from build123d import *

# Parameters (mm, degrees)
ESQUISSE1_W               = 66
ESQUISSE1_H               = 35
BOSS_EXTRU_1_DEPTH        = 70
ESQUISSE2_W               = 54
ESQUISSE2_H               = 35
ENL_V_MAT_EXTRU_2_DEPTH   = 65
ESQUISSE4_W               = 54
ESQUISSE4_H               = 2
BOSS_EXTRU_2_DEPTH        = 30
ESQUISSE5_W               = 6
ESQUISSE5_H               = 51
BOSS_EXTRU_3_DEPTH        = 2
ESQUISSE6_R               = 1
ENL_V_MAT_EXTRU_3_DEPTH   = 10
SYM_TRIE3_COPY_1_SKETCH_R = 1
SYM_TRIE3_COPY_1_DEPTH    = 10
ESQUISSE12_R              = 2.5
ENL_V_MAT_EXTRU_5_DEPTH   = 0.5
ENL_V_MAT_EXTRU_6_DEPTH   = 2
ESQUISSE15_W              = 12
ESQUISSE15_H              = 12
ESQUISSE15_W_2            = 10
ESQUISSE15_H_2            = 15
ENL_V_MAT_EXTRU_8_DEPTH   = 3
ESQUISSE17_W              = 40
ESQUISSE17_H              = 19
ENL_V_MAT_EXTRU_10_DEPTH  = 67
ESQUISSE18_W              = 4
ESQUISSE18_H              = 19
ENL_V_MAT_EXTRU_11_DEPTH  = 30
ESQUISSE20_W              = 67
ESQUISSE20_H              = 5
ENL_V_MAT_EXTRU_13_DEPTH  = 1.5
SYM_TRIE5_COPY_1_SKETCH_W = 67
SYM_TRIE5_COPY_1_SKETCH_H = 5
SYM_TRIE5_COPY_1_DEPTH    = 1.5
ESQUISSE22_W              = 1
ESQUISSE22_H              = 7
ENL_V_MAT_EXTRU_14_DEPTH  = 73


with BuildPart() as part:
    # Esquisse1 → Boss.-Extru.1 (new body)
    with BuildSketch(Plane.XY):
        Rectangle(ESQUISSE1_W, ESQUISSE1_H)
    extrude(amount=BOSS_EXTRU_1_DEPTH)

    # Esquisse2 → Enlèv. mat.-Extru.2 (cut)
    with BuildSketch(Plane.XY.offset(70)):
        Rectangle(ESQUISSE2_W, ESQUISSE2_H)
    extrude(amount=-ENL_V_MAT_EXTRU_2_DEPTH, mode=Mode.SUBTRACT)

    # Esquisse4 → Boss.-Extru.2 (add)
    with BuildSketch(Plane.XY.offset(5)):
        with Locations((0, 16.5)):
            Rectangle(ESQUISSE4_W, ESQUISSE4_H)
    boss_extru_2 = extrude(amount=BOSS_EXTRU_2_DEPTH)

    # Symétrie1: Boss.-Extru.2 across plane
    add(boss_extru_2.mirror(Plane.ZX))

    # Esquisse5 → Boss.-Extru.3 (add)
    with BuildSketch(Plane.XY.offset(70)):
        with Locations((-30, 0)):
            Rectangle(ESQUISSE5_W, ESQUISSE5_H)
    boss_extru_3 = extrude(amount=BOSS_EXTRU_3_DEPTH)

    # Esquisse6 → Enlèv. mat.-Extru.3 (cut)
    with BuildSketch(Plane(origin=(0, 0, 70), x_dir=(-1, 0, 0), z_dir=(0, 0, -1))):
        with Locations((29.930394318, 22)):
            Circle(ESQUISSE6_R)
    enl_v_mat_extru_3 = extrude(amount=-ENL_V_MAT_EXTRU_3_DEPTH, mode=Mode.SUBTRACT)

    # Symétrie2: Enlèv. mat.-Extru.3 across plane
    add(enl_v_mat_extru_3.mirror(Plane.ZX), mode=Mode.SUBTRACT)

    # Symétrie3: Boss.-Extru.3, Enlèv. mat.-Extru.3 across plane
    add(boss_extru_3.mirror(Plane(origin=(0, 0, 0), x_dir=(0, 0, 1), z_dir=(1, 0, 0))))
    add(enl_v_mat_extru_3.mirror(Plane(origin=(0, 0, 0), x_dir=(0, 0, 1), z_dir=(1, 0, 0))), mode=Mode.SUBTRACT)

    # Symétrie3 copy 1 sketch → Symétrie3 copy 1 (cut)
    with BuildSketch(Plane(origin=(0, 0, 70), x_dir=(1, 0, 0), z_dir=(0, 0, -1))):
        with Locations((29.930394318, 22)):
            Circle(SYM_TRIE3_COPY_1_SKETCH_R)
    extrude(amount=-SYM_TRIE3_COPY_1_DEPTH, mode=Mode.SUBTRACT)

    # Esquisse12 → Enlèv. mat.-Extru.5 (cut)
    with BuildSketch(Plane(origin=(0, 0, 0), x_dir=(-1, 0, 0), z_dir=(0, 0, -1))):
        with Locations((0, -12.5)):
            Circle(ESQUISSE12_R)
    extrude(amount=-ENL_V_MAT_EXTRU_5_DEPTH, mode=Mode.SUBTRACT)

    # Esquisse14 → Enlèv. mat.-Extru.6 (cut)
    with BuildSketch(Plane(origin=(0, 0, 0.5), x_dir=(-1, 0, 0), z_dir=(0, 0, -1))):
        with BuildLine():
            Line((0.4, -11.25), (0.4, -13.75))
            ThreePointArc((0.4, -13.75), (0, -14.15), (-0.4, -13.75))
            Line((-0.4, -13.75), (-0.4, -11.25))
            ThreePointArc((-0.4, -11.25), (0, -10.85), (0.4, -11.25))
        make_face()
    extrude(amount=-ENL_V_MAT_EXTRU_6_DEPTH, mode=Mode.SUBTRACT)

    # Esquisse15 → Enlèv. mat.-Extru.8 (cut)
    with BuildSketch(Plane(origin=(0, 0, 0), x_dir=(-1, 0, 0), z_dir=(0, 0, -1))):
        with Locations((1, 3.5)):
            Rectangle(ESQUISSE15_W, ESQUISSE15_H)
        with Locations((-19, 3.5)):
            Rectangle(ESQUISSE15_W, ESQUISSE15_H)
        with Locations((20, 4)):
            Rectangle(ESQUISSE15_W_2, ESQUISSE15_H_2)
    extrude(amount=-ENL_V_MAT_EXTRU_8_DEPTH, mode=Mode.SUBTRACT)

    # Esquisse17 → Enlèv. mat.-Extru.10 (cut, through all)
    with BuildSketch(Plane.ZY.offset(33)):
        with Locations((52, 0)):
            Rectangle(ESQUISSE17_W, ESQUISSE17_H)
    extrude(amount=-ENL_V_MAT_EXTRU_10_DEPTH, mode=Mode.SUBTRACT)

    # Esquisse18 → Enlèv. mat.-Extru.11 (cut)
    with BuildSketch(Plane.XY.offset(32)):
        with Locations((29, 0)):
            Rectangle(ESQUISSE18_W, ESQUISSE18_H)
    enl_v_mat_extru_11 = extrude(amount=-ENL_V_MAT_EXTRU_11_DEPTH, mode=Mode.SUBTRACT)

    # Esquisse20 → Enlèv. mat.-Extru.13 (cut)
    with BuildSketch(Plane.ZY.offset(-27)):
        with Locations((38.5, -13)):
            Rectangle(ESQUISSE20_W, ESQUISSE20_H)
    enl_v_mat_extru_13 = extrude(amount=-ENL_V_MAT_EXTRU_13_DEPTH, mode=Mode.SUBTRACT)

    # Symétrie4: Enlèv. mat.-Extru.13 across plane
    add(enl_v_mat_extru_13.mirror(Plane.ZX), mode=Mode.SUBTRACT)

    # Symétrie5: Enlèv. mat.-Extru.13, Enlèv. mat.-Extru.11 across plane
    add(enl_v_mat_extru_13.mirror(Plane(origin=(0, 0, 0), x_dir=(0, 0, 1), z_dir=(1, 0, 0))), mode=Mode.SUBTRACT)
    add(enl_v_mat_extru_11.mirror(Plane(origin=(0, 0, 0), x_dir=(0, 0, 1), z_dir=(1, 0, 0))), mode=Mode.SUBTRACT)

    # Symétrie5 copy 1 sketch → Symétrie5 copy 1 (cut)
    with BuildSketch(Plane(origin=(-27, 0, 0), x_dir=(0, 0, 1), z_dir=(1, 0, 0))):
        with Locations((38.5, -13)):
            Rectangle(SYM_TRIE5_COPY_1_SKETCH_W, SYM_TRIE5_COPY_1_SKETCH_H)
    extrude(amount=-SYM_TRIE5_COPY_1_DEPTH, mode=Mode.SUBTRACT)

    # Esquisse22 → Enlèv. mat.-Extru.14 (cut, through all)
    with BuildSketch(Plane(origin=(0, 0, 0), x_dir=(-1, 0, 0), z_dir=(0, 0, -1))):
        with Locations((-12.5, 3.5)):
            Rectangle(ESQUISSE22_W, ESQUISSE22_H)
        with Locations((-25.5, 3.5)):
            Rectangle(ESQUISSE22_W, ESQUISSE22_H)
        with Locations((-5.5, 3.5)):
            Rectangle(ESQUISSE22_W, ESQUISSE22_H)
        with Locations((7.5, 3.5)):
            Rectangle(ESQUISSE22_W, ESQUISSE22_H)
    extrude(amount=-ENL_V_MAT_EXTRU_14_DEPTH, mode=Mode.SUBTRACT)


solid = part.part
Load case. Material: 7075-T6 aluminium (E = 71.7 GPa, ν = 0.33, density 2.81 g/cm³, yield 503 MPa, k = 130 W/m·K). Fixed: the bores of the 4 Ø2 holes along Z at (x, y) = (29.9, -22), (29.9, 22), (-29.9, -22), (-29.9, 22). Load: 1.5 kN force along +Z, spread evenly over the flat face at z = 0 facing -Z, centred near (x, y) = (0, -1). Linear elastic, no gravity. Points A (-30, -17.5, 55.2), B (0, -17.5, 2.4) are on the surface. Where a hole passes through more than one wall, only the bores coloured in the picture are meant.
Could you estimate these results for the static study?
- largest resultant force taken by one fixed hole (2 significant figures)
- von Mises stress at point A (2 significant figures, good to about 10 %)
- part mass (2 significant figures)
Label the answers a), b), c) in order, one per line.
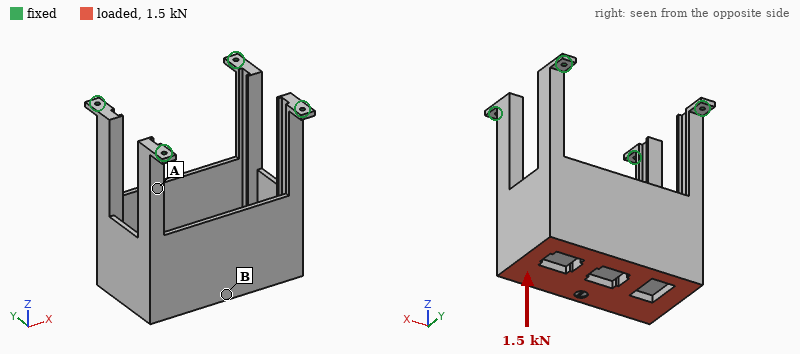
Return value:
a) 400 N
b) 27 MPa
c) 83 g
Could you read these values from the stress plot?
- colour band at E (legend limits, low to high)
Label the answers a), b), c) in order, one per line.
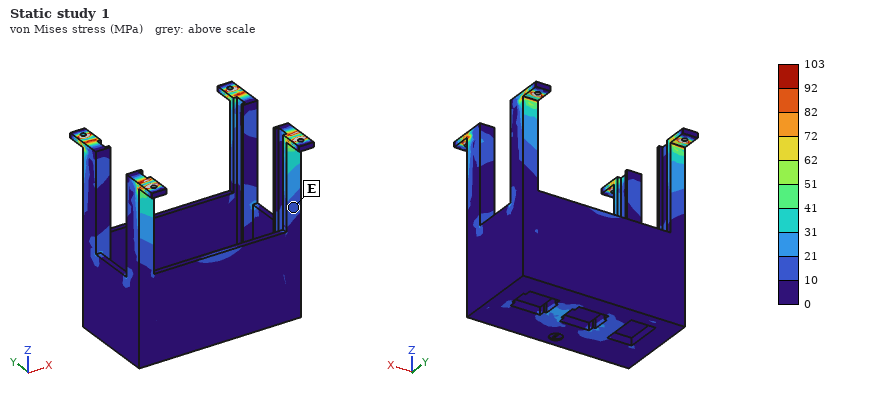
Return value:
a) 10 to 21 MPa
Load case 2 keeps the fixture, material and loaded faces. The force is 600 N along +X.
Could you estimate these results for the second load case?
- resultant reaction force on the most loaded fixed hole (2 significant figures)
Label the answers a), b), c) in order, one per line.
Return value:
a) 360 N
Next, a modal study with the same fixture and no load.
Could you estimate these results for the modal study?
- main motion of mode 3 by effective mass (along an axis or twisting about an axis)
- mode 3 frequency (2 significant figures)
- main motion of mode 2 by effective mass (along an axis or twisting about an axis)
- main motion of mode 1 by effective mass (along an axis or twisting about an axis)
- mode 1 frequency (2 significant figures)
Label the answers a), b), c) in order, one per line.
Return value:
a) twisting about Z
b) 1500 Hz
c) along Y
d) along X
e) 690 Hz
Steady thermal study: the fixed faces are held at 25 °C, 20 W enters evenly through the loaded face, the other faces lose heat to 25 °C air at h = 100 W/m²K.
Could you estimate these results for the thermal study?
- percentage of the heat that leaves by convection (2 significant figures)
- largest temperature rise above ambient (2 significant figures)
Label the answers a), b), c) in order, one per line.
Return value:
a) 90 %
b) 14 K
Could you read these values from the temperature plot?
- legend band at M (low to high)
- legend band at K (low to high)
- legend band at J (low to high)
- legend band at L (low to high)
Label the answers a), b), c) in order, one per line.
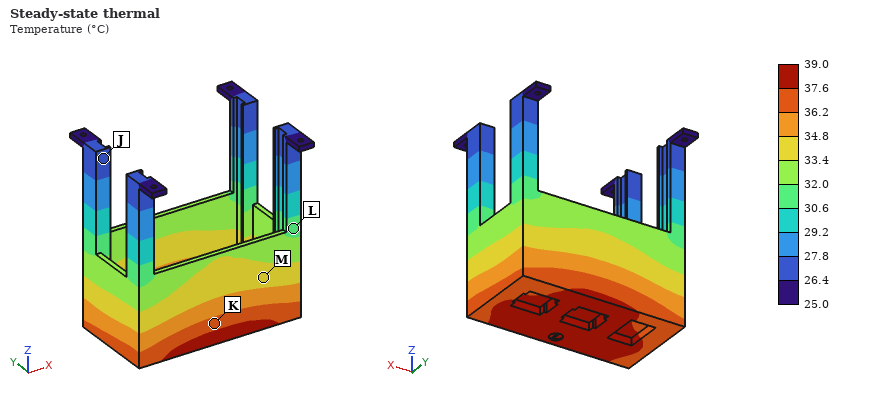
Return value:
a) 33.4 to 34.8 °C
b) 36.2 to 37.6 °C
c) 26.4 to 27.8 °C
d) 30.6 to 32.0 °C
